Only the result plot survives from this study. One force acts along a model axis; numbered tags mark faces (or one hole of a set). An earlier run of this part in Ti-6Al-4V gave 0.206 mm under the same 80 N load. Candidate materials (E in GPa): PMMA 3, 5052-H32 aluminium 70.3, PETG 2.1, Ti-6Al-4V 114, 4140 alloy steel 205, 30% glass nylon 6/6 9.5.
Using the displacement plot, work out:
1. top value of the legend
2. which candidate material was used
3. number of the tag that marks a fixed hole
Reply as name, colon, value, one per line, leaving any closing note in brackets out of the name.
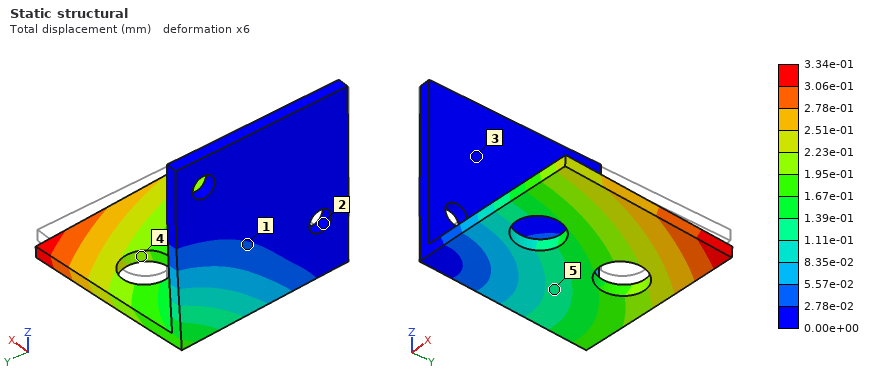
top value of the legend: 3.34e-01 mm
which candidate material was used: 5052-H32 aluminium
number of the tag that marks a fixed hole: 2
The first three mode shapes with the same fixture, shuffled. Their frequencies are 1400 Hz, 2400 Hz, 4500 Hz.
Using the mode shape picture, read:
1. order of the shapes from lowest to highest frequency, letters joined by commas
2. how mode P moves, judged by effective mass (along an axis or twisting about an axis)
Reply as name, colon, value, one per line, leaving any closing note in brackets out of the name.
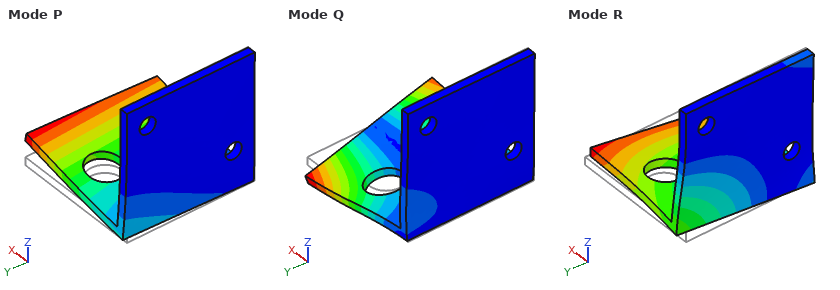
order of the shapes from lowest to highest frequency, letters joined by commas: P, R, Q
how mode P moves, judged by effective mass: along Z
